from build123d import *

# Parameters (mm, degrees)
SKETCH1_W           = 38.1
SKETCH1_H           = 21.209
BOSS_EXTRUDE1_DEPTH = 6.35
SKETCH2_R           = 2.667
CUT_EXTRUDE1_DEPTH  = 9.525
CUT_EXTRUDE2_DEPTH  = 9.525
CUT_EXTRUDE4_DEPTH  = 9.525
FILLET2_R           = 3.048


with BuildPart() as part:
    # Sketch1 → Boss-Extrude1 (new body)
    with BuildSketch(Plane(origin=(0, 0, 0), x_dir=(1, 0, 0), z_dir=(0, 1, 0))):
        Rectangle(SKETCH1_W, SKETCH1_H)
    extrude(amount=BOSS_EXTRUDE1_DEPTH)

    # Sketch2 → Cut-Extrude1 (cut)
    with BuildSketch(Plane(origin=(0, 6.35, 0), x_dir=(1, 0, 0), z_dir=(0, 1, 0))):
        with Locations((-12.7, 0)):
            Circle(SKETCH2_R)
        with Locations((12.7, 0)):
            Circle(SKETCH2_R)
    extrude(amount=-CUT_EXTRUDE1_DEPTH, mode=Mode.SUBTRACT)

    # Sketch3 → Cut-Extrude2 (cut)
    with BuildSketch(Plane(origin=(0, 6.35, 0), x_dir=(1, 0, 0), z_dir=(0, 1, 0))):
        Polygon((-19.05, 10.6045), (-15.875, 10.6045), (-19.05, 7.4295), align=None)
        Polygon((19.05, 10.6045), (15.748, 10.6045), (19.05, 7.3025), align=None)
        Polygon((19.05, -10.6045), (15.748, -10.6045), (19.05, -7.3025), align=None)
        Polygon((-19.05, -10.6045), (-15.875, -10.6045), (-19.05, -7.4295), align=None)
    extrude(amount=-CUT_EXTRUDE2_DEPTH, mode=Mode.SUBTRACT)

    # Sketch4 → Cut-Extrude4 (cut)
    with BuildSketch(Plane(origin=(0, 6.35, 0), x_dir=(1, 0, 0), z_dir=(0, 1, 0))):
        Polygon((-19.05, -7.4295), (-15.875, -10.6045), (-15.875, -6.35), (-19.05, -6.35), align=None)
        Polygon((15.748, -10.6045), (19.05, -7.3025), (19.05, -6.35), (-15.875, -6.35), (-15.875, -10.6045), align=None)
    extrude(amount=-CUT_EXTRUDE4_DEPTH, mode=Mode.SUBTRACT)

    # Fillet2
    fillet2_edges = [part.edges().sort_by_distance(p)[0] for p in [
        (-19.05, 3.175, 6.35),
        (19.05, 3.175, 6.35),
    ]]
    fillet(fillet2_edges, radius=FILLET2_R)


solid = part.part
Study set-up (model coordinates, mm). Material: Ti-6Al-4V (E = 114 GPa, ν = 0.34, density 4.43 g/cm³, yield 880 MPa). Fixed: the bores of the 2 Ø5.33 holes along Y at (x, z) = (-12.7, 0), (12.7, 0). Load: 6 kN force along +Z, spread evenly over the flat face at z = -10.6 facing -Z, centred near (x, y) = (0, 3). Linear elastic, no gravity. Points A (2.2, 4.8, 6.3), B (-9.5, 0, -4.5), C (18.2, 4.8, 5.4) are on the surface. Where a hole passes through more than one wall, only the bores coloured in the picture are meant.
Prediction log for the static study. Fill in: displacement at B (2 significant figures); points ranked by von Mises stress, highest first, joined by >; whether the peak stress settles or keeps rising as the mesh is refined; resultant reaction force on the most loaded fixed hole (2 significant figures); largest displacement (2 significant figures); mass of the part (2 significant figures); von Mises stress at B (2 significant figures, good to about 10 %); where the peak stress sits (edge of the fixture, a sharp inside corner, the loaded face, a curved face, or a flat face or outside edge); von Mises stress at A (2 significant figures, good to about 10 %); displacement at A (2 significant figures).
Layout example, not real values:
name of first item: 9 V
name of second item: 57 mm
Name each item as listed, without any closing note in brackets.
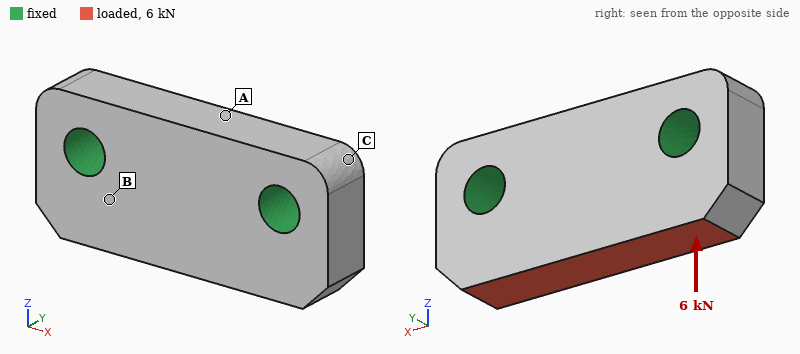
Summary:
displacement at B: 1.9 µm
points ranked by von Mises stress, highest first, joined by >: B > A > C
whether the peak stress settles or keeps rising as the mesh is refined: keeps rising
resultant reaction force on the most loaded fixed hole: 3.1 kN
largest displacement: 5.7 µm
mass of the part: 17 g
von Mises stress at B: 46 MPa
where the peak stress sits: edge of the fixture
von Mises stress at A: 27 MPa
displacement at A: 3.6 µm
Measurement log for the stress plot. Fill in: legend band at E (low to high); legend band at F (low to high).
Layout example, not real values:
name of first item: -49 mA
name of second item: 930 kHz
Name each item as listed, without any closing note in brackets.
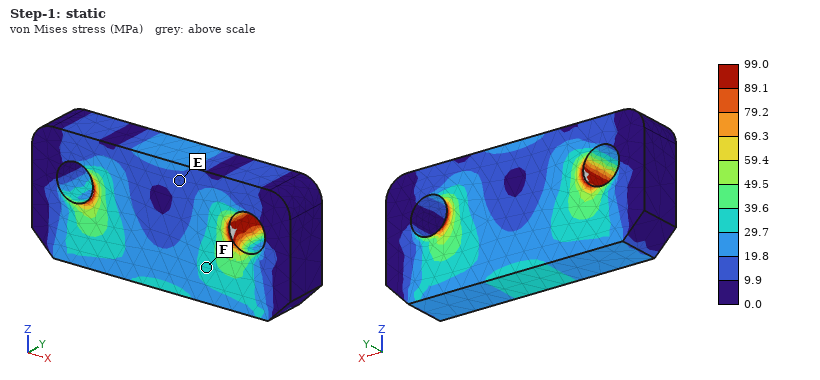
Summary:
legend band at E: 9.9 to 19.8 MPa
legend band at F: 29.7 to 39.6 MPa
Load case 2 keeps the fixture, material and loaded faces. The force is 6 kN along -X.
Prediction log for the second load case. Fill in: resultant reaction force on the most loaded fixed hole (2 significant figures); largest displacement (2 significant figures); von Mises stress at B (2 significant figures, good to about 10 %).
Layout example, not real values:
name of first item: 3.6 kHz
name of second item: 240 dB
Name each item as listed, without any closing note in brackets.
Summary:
resultant reaction force on the most loaded fixed hole: 3.6 kN
largest displacement: 8.8 µm
von Mises stress at B: 58 MPa
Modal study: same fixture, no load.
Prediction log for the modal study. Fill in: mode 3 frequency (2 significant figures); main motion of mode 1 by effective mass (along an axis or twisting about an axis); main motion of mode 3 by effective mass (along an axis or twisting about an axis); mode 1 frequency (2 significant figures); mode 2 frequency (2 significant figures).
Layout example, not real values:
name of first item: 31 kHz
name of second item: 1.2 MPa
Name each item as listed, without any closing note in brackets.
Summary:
mode 3 frequency: 51 kHz
main motion of mode 1 by effective mass: along Y
main motion of mode 3 by effective mass: along Z
mode 1 frequency: 33 kHz
mode 2 frequency: 47 kHz
